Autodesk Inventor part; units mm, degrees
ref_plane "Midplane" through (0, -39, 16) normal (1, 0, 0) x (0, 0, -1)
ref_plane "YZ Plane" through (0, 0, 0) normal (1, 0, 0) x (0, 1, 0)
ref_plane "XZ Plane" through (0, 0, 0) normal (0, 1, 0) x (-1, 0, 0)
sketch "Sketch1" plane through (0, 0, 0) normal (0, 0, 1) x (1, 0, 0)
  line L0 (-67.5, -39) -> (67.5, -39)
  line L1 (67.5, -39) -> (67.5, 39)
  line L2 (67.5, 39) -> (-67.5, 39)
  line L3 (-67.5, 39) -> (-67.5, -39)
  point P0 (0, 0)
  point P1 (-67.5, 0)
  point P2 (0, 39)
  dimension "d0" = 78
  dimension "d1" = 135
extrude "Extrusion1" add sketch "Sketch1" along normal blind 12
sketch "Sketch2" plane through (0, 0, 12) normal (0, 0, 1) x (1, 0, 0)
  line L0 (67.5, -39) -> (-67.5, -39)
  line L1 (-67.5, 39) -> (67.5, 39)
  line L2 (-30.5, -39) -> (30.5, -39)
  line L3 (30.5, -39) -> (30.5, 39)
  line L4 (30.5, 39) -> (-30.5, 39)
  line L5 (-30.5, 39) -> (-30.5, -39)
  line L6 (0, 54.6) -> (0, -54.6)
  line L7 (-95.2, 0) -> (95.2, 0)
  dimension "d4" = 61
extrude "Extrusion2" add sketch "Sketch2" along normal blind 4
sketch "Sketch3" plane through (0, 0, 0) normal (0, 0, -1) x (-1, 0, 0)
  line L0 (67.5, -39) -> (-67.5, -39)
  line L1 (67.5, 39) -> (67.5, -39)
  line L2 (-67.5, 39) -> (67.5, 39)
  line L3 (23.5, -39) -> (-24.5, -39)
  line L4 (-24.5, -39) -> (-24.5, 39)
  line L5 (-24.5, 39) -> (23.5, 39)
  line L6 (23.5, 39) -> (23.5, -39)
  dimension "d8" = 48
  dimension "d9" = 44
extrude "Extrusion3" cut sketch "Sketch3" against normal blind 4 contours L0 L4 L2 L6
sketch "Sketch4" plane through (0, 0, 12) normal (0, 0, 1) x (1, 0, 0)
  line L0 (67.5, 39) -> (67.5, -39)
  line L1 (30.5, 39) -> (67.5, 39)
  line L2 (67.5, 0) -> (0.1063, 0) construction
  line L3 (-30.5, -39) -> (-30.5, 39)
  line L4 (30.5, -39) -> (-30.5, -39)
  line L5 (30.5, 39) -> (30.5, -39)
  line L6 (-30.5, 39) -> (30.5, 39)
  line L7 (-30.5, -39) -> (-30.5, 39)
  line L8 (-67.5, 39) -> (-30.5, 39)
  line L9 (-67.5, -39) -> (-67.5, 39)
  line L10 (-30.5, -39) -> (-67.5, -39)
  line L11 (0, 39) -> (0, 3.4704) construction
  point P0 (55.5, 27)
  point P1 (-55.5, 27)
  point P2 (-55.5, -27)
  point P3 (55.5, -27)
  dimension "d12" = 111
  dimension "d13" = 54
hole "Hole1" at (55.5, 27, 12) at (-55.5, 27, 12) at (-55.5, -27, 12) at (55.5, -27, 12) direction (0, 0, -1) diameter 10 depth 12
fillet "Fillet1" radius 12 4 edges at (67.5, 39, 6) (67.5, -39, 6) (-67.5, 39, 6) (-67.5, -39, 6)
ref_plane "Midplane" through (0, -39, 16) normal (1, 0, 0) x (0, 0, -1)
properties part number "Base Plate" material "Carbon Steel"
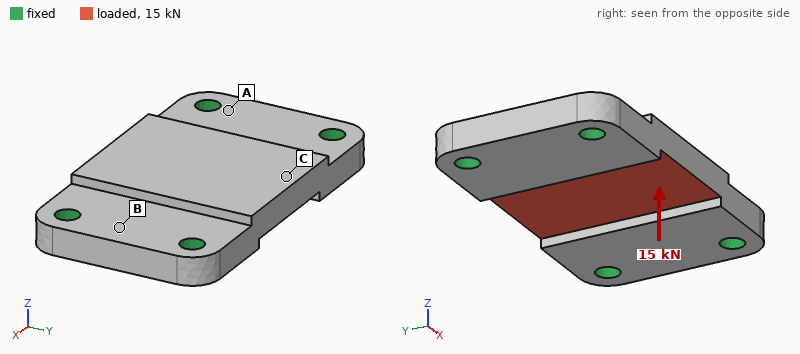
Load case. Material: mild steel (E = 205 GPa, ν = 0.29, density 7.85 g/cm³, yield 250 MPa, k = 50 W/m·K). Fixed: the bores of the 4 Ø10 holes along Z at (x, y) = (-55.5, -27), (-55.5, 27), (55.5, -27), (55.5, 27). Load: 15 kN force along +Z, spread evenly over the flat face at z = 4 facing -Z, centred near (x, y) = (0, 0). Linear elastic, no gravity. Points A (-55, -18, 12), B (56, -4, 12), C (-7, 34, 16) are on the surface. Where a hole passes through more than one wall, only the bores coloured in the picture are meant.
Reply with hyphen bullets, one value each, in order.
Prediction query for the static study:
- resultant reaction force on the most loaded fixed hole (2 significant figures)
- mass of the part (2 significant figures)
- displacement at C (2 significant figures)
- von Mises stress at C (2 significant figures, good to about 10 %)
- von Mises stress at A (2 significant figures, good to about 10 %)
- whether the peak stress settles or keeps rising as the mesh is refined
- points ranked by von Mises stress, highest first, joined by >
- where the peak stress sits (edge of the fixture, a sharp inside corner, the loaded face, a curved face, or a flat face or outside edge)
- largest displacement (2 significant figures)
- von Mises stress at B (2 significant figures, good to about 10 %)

- 6.4 kN
- 980 g
- 36 µm
- 68 MPa
- 33 MPa
- keeps rising
- C > A > B
- edge of the fixture
- 39 µm
- 17 MPa
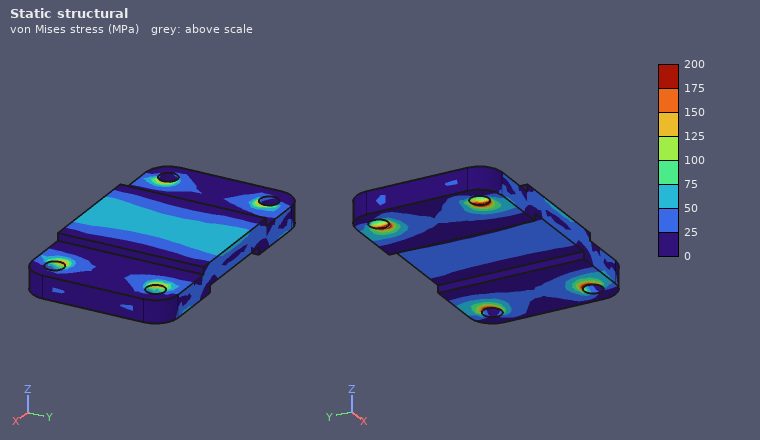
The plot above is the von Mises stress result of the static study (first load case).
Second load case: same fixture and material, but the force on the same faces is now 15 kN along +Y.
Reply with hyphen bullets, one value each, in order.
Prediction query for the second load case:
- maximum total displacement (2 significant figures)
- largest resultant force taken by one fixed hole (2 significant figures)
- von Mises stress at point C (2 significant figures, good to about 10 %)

- 9.2 µm
- 4.6 kN
- 19 MPa
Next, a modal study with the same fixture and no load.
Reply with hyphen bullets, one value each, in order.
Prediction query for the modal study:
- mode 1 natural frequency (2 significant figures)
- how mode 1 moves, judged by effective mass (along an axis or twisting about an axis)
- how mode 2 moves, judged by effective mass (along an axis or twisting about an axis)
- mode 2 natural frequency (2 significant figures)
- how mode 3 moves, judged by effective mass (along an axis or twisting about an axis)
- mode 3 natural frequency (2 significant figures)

- 5100 Hz
- along Z
- twisting about X
- 6900 Hz
- twisting about Y
- 11 kHz
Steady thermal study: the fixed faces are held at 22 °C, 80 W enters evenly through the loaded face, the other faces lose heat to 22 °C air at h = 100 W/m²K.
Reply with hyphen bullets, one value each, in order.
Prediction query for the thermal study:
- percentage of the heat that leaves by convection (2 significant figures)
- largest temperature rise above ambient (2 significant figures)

- 34 %
- 31 K
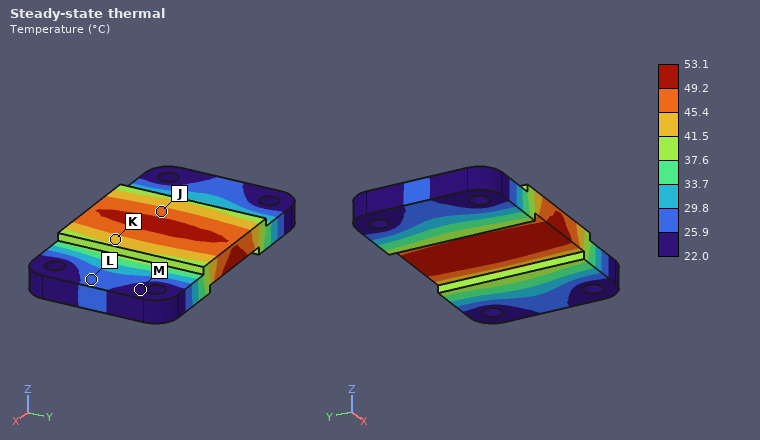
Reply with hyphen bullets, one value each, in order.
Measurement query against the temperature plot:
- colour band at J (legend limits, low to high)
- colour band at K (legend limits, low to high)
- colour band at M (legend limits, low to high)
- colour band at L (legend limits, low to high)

- 45.4 to 49.2 °C
- 41.5 to 45.4 °C
- 22.0 to 25.9 °C
- 25.9 to 29.8 °C
